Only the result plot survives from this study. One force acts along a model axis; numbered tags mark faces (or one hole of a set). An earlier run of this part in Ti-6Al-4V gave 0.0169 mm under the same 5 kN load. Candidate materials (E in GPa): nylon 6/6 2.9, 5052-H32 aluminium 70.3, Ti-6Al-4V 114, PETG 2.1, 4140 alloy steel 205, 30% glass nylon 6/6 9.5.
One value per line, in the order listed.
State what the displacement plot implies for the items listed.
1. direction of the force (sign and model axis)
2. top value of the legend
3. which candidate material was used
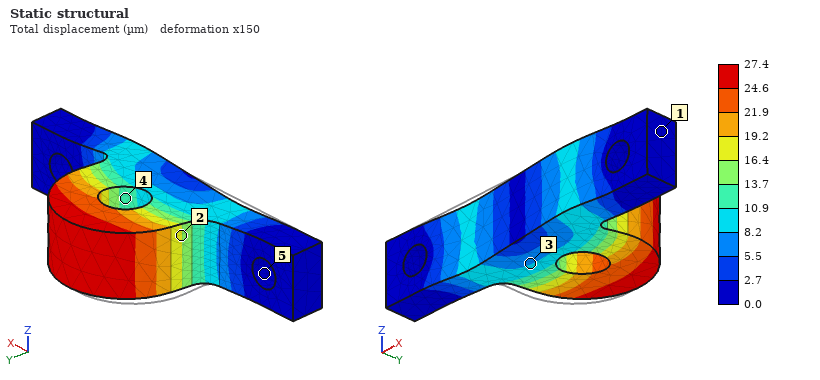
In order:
+X
27.4 µm
5052-H32 aluminium
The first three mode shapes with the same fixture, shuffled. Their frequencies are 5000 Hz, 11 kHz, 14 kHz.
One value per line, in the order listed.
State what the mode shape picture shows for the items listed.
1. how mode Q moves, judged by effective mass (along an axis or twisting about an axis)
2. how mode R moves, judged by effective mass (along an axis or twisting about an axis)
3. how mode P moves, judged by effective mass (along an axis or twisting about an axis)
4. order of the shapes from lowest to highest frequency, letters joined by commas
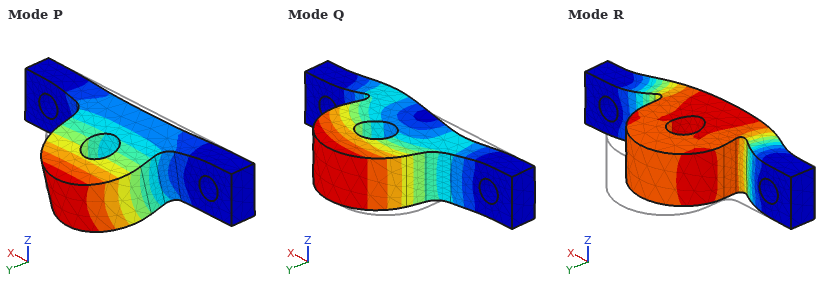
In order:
along X
along Y
along Z
P, R, Q
